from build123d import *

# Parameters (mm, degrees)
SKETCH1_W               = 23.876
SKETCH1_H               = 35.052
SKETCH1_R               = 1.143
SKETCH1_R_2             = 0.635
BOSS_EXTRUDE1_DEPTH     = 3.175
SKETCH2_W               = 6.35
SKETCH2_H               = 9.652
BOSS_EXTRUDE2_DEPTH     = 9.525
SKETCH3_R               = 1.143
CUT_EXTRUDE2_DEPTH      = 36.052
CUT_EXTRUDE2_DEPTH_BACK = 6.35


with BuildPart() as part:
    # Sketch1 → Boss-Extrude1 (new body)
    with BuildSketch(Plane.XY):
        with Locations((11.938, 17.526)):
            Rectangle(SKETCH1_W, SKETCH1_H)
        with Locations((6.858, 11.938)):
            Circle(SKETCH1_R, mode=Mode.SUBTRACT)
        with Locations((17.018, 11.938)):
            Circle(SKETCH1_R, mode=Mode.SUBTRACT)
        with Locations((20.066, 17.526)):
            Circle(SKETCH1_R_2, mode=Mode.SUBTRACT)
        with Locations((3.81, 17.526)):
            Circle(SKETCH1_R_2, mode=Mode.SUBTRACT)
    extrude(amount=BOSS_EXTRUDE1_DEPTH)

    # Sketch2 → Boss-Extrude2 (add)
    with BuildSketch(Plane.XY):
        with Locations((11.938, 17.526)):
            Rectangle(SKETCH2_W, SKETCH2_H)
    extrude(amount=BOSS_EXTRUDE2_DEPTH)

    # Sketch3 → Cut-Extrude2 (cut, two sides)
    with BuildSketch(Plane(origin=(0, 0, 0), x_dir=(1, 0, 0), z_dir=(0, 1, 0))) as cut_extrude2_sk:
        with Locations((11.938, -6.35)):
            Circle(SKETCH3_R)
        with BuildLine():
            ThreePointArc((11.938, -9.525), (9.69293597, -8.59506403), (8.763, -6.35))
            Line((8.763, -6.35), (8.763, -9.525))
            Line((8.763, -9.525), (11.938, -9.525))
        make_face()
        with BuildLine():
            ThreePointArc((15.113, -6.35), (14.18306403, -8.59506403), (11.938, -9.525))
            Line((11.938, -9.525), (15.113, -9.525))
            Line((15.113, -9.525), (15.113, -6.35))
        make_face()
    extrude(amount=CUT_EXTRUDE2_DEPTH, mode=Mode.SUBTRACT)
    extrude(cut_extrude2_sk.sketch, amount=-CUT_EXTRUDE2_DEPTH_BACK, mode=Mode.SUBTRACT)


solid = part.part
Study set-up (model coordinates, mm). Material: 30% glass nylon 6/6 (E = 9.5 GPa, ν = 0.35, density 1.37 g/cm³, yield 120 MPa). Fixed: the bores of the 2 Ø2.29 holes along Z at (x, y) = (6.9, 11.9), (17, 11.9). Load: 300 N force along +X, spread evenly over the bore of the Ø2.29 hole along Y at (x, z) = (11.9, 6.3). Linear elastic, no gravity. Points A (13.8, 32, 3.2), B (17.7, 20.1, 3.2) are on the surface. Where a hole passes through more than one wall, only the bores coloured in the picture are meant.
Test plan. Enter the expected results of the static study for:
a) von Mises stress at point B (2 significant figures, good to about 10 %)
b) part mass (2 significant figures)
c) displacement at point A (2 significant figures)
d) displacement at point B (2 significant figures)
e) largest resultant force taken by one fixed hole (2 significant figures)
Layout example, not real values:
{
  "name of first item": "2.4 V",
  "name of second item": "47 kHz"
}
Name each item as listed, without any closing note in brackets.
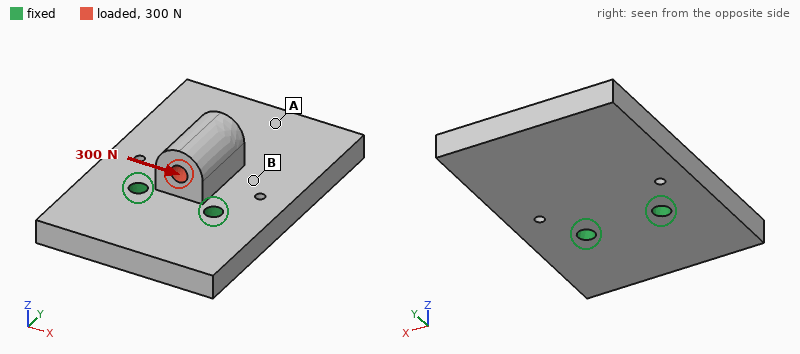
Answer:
{
  "von Mises stress at point B": "7.3 MPa",
  "part mass": "4.0 g",
  "displacement at point A": "20 µm",
  "displacement at point B": "19 µm",
  "largest resultant force taken by one fixed hole": "250 N"
}
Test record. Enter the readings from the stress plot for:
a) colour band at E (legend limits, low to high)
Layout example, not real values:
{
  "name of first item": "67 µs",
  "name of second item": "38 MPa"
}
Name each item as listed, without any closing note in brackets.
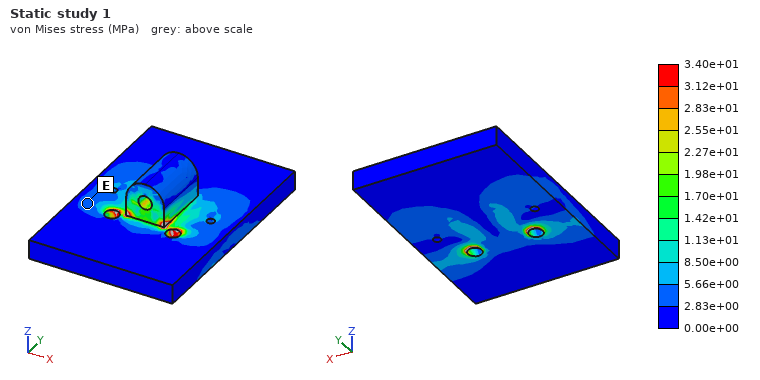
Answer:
{
  "colour band at E": "2.83e+00 to 5.66e+00 MPa"
}
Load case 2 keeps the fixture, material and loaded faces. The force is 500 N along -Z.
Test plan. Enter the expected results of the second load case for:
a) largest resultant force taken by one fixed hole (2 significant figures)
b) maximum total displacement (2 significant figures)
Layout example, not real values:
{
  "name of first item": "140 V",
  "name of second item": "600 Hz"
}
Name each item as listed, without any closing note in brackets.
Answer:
{
  "largest resultant force taken by one fixed hole": "250 N",
  "maximum total displacement": "0.35 mm"
}
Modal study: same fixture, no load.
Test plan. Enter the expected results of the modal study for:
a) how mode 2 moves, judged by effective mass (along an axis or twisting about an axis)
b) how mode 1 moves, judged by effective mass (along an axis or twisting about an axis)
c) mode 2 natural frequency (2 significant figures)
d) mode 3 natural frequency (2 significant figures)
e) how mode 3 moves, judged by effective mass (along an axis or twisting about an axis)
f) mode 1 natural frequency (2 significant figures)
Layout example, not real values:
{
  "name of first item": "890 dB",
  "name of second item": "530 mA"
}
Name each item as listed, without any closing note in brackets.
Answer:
{
  "how mode 2 moves, judged by effective mass": "twisting about Y",
  "how mode 1 moves, judged by effective mass": "along Z",
  "mode 2 natural frequency": "5900 Hz",
  "mode 3 natural frequency": "8800 Hz",
  "how mode 3 moves, judged by effective mass": "along Z",
  "mode 1 natural frequency": "2700 Hz"
}
